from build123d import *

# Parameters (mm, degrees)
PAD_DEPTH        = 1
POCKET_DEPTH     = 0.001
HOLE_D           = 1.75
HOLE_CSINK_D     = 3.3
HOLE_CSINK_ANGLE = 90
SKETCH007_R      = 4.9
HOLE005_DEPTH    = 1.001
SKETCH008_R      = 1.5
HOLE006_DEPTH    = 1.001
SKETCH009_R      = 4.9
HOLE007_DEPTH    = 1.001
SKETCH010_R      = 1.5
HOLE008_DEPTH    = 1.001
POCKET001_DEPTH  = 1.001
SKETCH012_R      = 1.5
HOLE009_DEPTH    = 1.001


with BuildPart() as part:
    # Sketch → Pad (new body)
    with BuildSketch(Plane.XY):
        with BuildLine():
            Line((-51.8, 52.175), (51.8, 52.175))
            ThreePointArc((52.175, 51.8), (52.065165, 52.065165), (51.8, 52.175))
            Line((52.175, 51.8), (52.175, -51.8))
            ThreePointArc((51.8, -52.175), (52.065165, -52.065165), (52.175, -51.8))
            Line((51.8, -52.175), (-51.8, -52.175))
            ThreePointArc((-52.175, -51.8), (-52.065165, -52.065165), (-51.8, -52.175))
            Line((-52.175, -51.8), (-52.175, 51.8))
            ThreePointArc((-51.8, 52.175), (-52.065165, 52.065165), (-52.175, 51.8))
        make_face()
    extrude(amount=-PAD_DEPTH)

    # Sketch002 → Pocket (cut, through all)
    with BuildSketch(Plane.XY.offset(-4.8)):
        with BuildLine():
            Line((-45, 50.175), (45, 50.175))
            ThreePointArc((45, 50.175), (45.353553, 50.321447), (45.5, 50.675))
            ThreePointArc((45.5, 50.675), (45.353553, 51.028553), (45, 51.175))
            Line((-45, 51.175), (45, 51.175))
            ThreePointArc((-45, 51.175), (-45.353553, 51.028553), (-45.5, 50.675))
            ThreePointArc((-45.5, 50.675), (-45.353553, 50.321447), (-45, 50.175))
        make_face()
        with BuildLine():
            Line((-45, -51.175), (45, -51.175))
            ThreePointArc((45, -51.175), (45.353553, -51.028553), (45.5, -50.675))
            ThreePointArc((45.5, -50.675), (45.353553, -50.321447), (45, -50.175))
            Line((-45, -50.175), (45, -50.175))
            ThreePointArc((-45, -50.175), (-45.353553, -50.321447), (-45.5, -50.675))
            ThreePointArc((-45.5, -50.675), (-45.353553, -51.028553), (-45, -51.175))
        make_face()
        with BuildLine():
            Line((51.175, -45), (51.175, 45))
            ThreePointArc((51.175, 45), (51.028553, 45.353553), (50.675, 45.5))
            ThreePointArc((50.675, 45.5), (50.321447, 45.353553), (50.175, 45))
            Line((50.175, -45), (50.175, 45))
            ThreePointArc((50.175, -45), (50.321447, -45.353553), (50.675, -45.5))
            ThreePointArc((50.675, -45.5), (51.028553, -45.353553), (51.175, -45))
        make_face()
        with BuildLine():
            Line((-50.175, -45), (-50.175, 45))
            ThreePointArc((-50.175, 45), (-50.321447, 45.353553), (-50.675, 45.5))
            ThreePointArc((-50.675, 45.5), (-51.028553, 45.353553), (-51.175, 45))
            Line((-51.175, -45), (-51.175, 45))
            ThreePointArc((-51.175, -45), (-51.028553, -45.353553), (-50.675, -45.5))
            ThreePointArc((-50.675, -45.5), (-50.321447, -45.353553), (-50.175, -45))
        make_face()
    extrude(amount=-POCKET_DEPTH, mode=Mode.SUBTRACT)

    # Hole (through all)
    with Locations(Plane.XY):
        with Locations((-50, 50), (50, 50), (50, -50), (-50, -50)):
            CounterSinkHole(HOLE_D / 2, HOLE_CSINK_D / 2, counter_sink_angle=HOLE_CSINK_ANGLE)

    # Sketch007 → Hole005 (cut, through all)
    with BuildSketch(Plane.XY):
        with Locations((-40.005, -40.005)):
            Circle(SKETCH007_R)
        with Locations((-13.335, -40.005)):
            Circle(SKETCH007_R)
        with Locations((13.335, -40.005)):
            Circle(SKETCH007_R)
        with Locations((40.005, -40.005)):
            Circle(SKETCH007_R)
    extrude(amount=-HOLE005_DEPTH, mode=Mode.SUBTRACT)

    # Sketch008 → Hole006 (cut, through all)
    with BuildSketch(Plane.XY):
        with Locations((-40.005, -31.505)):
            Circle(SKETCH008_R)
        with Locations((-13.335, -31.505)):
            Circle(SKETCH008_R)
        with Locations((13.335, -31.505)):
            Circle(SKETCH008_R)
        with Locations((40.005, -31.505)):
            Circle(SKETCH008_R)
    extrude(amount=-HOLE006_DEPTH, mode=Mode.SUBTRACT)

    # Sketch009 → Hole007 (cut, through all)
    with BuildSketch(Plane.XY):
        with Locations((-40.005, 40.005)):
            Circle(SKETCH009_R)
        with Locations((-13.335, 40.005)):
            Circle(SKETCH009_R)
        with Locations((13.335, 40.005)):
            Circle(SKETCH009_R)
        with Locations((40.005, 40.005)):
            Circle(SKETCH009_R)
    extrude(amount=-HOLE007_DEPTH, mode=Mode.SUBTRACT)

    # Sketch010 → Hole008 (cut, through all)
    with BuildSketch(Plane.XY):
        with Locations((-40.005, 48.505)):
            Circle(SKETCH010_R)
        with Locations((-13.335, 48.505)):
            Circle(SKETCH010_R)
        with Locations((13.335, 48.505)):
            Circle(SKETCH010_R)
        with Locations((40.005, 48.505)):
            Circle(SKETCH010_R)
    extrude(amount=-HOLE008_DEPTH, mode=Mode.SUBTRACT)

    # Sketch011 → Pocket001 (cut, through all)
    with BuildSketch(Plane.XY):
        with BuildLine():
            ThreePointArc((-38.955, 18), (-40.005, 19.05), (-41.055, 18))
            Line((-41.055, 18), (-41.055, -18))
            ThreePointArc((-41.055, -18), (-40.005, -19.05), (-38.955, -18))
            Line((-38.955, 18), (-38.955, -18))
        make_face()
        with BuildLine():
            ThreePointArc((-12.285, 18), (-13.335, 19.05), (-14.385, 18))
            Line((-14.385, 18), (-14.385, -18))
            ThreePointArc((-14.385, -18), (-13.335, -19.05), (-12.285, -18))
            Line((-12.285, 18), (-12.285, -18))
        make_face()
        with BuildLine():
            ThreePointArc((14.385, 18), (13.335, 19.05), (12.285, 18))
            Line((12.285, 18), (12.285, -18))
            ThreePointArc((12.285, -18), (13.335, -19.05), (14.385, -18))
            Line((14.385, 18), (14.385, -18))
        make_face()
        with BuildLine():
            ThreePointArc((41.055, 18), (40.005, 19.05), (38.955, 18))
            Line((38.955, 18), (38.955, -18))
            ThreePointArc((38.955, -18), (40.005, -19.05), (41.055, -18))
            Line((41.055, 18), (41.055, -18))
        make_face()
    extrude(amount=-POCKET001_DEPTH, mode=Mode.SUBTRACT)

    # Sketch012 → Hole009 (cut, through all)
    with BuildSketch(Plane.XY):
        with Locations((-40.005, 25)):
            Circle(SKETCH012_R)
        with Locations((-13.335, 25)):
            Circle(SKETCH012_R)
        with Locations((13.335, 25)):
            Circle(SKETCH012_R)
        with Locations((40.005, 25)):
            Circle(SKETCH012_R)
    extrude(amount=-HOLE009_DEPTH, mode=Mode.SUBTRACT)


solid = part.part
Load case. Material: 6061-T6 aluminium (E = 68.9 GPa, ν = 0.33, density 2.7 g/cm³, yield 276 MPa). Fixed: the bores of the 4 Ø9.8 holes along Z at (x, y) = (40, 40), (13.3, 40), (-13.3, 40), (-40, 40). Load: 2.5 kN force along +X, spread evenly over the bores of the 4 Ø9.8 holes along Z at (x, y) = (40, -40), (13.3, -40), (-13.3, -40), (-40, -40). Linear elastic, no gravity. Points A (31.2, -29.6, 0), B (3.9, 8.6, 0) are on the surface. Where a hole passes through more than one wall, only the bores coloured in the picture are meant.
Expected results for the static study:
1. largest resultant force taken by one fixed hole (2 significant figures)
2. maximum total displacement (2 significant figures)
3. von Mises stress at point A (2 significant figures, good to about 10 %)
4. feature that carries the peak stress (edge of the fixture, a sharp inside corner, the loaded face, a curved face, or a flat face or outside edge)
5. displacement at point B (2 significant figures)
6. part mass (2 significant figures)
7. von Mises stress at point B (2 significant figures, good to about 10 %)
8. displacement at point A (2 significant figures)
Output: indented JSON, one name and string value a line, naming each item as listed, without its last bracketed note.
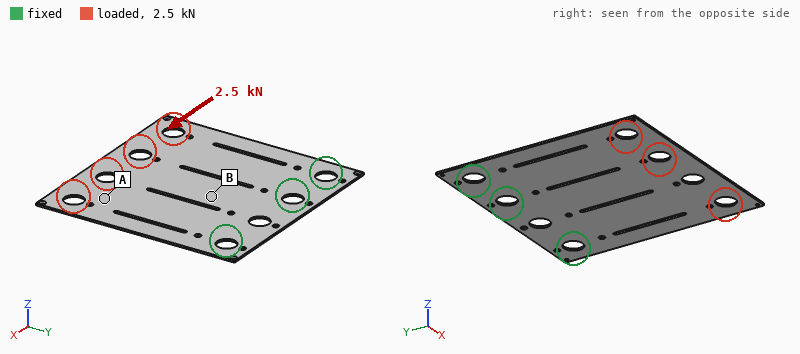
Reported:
{
  "largest resultant force taken by one fixed hole": "2.2 kN",
  "maximum total displacement": "0.28 mm",
  "von Mises stress at point A": "26 MPa",
  "feature that carries the peak stress": "a curved face",
  "displacement at point B": "0.064 mm",
  "part mass": "27 g",
  "von Mises stress at point B": "84 MPa",
  "displacement at point A": "0.22 mm"
}
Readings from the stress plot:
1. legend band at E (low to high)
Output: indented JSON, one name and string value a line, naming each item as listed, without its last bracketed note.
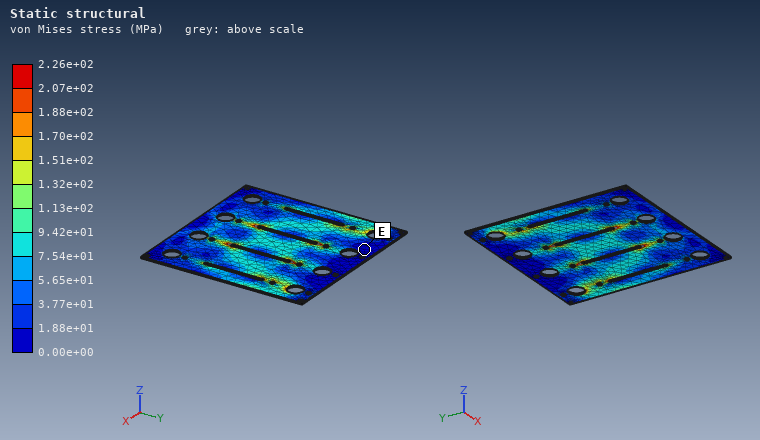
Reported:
{
  "legend band at E": "0.00e+00 to 1.88e+01 MPa"
}
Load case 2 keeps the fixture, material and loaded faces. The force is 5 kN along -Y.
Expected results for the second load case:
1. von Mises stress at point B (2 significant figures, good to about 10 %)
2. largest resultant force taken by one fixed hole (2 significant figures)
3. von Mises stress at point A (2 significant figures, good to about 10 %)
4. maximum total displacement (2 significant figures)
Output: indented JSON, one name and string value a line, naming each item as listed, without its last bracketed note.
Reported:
{
  "von Mises stress at point B": "53 MPa",
  "largest resultant force taken by one fixed hole": "1.3 kN",
  "von Mises stress at point A": "49 MPa",
  "maximum total displacement": "70 µm"
}
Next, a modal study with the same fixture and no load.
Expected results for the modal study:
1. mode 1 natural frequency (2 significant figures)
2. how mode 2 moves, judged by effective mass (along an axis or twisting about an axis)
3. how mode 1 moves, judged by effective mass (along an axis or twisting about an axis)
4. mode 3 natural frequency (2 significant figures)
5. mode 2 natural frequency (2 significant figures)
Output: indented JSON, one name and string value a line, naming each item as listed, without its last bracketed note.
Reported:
{
  "mode 1 natural frequency": "110 Hz",
  "how mode 2 moves, judged by effective mass": "twisting about Y",
  "how mode 1 moves, judged by effective mass": "along Z",
  "mode 3 natural frequency": "570 Hz",
  "mode 2 natural frequency": "230 Hz"
}
